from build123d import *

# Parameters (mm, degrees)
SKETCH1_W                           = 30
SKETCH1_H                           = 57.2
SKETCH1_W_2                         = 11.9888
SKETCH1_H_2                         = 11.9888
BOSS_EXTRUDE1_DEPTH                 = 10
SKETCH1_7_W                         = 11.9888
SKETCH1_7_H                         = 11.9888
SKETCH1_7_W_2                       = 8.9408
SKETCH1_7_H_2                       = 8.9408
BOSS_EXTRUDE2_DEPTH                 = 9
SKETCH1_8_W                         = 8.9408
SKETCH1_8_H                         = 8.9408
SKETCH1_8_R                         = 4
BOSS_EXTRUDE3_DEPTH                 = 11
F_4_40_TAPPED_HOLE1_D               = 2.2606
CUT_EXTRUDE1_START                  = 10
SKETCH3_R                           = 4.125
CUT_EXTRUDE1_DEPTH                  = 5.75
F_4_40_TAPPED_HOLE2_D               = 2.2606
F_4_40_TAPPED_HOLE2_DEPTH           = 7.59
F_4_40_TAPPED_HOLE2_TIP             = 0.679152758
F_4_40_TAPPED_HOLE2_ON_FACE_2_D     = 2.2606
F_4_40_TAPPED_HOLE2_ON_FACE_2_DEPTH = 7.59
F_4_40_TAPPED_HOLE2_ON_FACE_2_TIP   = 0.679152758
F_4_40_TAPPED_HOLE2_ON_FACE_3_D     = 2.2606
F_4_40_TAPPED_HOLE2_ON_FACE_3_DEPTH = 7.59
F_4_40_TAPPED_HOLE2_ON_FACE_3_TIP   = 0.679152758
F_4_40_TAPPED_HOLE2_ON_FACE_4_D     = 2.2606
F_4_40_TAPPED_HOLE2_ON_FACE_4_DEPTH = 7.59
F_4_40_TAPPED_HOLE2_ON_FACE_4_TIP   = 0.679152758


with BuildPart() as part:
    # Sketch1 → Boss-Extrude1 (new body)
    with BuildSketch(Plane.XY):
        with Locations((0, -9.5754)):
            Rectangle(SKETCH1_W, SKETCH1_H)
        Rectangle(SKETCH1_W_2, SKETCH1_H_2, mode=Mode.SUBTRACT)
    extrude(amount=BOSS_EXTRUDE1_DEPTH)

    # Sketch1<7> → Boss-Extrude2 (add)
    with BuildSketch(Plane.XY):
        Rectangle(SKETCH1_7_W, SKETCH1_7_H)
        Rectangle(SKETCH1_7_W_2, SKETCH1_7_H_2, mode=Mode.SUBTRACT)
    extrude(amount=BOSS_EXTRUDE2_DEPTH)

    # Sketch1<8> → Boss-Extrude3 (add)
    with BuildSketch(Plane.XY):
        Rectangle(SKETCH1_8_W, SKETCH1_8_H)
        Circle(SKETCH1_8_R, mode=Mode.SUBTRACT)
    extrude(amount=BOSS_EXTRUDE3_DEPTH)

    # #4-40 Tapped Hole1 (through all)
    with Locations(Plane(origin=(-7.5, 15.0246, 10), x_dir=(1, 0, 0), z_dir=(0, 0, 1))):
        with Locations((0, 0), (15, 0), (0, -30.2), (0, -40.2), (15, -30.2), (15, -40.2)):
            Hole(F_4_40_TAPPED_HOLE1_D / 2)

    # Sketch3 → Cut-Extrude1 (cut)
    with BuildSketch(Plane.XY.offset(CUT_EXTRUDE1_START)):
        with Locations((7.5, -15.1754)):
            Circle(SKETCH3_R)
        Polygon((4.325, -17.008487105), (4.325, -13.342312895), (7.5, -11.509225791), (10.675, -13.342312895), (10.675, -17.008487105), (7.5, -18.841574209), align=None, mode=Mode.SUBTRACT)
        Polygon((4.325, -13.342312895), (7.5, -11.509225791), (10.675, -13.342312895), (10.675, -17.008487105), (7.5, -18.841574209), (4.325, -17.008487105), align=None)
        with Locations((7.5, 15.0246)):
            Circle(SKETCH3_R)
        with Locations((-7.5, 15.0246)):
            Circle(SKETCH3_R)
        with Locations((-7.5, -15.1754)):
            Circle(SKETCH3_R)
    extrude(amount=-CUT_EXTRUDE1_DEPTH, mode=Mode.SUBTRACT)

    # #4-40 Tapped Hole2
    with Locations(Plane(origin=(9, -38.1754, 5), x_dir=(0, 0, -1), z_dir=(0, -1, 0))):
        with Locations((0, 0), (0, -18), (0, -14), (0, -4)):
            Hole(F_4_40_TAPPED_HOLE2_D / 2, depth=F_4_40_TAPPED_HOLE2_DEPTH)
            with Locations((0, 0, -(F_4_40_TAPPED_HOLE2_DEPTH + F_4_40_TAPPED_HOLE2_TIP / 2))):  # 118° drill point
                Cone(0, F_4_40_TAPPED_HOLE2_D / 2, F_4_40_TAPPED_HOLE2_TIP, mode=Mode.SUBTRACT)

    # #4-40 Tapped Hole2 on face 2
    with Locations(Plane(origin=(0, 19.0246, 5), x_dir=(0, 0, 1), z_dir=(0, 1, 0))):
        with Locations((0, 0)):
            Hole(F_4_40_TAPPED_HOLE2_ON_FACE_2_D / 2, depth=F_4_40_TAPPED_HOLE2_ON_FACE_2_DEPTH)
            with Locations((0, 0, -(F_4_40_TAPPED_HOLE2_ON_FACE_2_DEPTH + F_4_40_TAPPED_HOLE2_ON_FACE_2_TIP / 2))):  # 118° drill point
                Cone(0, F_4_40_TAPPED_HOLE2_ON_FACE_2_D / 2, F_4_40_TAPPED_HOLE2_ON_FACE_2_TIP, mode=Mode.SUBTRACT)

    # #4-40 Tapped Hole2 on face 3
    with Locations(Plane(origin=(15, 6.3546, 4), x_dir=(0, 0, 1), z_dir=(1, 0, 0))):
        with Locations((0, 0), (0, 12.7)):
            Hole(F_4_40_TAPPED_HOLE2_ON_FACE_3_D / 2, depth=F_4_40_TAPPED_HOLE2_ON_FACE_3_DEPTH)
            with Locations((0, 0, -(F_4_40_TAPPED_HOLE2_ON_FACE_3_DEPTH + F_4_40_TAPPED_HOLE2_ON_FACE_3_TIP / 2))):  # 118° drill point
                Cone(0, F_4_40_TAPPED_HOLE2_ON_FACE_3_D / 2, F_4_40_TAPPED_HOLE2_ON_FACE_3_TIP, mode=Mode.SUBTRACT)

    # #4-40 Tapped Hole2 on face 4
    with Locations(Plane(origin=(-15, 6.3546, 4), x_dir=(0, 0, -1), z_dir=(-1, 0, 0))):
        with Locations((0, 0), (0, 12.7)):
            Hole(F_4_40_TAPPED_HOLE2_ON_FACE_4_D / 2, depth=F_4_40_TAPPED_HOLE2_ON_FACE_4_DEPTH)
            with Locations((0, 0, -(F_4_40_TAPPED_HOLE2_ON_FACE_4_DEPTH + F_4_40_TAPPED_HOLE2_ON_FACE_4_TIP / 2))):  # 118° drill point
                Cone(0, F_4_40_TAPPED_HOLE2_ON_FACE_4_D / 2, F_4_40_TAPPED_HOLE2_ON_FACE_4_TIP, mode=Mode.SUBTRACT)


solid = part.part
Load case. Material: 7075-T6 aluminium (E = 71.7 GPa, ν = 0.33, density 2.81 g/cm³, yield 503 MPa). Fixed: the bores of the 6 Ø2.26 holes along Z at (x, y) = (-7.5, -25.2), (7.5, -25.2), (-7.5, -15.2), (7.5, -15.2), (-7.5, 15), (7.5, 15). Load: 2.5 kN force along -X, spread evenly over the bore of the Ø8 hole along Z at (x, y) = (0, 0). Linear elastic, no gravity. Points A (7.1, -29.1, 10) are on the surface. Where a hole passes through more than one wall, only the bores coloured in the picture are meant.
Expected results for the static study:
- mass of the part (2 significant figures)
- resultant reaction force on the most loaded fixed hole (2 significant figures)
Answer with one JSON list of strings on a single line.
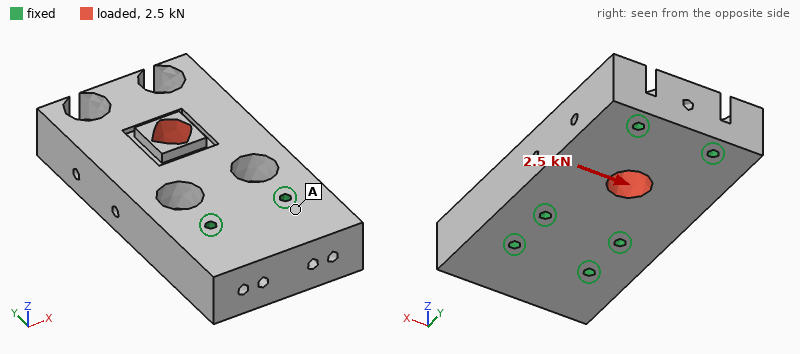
["42 g", "690 N"]
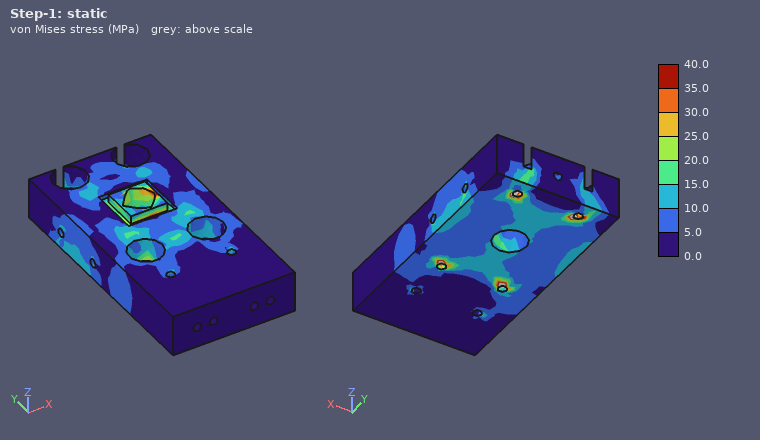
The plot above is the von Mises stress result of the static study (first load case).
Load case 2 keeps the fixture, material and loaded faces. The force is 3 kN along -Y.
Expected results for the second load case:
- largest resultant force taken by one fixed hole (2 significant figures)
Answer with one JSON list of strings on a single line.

["650 N"]
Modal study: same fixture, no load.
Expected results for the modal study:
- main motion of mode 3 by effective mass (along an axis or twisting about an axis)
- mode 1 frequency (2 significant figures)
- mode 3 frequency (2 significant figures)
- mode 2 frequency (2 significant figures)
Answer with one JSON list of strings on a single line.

["along Z", "23 kHz", "30 kHz", "23 kHz"]
